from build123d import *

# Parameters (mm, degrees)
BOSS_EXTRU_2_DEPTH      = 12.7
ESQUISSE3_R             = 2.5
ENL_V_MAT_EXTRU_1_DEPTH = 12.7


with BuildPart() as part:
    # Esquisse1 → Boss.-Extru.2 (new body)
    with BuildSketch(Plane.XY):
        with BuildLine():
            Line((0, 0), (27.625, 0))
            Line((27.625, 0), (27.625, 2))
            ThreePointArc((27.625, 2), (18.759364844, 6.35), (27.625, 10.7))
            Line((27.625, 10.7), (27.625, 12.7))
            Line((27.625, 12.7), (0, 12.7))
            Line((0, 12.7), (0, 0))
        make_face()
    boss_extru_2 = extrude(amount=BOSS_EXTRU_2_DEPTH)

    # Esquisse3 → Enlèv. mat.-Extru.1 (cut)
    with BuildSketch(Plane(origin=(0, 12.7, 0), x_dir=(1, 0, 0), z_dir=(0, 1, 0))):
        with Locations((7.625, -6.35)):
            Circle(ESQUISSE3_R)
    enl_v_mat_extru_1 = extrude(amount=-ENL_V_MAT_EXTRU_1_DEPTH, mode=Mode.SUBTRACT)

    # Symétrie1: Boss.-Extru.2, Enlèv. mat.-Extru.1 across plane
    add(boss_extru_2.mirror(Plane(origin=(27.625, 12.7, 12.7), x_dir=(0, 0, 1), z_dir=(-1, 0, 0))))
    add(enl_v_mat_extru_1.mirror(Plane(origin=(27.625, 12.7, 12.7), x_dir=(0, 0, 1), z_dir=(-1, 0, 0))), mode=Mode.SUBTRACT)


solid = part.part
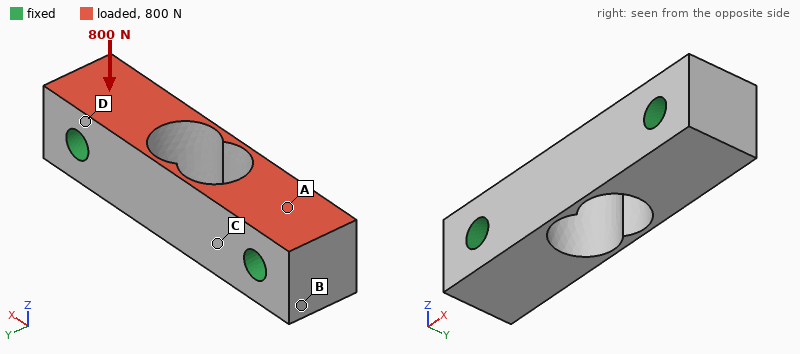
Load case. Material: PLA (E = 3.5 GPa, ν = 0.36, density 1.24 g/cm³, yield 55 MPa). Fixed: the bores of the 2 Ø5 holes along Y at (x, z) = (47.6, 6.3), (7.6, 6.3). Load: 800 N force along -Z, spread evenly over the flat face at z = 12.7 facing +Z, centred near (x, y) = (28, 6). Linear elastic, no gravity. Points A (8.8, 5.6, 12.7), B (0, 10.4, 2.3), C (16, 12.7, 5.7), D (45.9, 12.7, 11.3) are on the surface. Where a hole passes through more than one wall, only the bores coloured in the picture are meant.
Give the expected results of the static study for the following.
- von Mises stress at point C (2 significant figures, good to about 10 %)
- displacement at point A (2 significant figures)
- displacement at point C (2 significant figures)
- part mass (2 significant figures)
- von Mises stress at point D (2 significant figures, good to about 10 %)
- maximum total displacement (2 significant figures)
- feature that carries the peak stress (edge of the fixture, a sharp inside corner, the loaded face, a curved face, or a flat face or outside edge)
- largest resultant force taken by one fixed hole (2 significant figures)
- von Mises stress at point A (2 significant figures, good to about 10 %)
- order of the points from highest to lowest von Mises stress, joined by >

2.2 MPa
6.3 µm
14 µm
7.8 g
2.9 MPa
32 µm
edge of the fixture
400 N
4.4 MPa
A > D > C > B
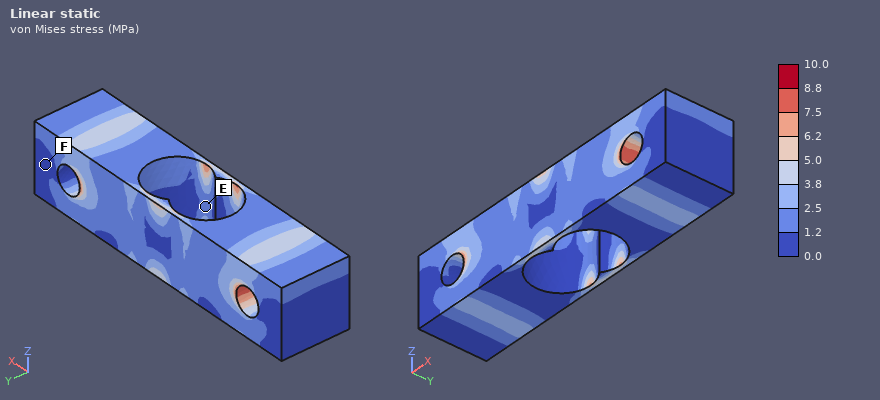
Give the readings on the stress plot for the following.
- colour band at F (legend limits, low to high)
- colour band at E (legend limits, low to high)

0.0 to 1.2 MPa
1.2 to 2.5 MPa
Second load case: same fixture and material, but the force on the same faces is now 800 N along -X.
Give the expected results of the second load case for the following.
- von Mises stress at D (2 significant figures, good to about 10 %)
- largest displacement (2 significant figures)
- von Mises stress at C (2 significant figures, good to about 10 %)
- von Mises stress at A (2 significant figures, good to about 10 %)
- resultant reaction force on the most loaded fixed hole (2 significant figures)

3.4 MPa
19 µm
1.2 MPa
2.6 MPa
400 N
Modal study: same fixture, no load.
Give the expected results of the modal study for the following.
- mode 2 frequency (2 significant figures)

10 kHz
